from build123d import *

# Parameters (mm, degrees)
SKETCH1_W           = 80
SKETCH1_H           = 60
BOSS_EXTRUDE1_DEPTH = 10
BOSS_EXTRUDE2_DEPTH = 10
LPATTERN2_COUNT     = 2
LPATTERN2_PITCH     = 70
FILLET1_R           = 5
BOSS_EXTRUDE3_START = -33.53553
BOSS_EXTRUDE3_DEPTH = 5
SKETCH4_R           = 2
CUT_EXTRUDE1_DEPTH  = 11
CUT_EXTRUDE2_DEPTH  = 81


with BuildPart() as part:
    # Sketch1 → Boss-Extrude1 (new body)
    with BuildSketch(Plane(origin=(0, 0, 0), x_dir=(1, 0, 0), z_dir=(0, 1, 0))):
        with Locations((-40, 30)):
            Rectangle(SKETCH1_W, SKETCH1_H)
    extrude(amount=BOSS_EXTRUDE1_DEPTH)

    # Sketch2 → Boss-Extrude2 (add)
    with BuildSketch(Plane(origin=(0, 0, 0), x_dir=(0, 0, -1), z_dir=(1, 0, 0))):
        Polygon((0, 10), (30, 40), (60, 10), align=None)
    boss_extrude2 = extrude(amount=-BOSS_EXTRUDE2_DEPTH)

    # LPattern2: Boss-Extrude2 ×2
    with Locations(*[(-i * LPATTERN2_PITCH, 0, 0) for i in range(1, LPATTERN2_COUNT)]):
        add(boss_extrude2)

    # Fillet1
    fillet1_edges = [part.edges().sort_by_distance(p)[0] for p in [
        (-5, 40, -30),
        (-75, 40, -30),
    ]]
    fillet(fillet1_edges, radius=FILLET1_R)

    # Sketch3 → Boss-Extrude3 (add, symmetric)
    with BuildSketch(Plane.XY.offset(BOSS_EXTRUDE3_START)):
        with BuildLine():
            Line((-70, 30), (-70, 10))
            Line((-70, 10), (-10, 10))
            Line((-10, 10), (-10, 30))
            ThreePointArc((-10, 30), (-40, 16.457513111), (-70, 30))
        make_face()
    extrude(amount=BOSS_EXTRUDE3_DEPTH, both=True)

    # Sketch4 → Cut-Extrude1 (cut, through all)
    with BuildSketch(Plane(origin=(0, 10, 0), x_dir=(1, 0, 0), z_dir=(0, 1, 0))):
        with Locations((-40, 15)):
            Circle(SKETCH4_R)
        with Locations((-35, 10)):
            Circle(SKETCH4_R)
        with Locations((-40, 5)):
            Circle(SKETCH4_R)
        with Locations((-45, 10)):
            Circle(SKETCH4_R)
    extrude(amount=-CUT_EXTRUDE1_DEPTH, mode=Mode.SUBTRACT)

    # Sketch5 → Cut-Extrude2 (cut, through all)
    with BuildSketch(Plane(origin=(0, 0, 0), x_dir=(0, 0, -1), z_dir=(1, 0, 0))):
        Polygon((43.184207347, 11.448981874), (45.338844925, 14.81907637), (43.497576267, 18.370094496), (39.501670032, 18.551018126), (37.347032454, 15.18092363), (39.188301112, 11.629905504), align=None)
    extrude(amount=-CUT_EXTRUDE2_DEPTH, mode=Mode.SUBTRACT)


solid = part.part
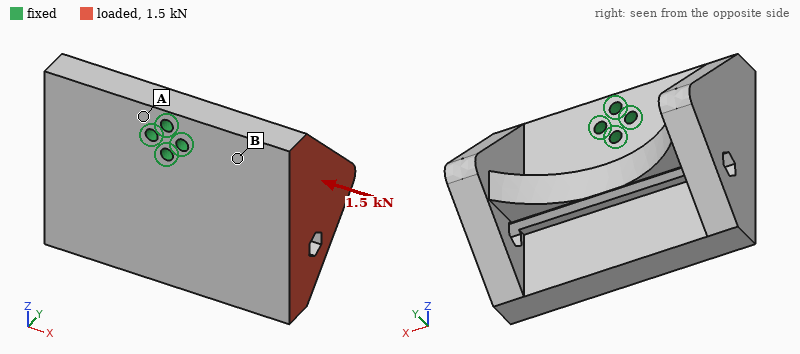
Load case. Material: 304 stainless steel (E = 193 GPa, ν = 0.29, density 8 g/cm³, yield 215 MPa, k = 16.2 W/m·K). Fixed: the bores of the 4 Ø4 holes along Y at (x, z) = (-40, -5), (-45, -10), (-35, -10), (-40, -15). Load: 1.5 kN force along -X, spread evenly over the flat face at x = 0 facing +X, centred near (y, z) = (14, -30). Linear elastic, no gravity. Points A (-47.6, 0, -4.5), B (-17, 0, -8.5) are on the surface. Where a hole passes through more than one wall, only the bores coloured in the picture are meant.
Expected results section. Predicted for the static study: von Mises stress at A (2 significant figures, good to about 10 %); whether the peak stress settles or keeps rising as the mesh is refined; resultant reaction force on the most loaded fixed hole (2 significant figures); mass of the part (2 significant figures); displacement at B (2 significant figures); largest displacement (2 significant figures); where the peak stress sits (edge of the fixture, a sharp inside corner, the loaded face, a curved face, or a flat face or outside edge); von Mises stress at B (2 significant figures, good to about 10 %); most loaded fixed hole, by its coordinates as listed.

14 MPa
keeps rising
1.8 kN
570 g
3.5 µm
15 µm
edge of the fixture
5.6 MPa
(-40, -15)
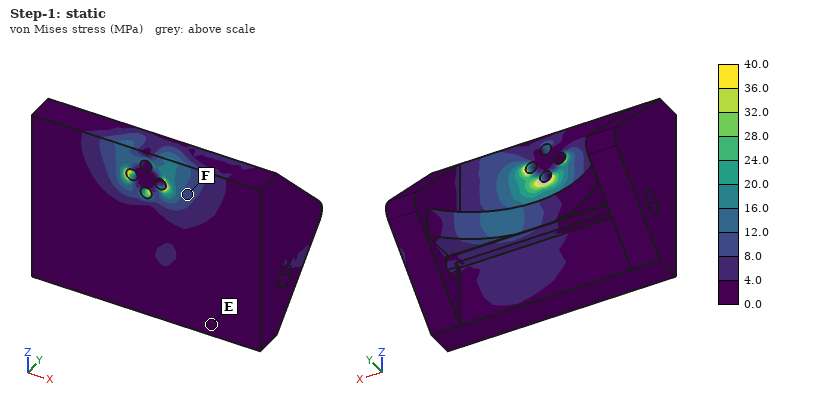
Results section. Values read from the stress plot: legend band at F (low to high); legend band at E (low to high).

8.0 to 12.0 MPa
0.0 to 4.0 MPa
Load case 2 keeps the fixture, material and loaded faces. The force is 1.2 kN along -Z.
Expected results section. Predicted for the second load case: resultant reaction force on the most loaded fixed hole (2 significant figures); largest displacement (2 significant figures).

2.2 kN
16 µm
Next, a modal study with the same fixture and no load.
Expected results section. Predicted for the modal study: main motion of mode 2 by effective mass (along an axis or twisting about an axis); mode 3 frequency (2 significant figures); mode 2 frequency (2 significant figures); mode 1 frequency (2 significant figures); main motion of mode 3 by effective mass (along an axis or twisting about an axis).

along Y
3200 Hz
2300 Hz
2200 Hz
along X
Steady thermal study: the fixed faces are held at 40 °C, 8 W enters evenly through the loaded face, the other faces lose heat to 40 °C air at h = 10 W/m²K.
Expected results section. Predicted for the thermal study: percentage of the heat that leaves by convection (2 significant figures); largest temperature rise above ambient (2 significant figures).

26 %
34 K
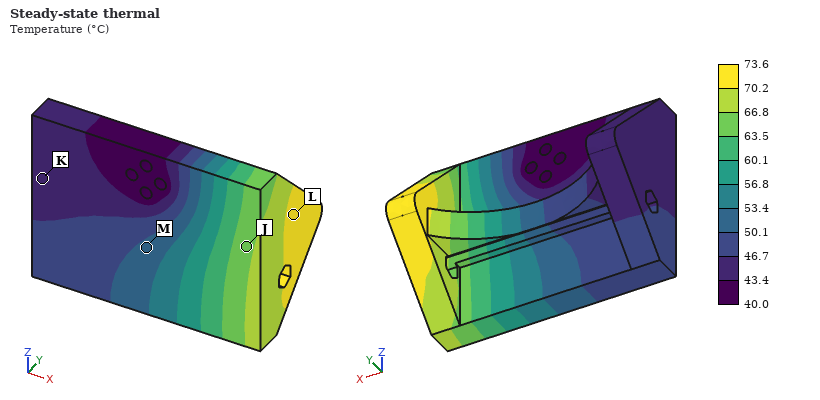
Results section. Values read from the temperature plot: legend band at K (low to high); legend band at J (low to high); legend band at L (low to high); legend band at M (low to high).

43.4 to 46.7 °C
63.5 to 66.8 °C
70.2 to 73.6 °C
50.1 to 53.4 °C
